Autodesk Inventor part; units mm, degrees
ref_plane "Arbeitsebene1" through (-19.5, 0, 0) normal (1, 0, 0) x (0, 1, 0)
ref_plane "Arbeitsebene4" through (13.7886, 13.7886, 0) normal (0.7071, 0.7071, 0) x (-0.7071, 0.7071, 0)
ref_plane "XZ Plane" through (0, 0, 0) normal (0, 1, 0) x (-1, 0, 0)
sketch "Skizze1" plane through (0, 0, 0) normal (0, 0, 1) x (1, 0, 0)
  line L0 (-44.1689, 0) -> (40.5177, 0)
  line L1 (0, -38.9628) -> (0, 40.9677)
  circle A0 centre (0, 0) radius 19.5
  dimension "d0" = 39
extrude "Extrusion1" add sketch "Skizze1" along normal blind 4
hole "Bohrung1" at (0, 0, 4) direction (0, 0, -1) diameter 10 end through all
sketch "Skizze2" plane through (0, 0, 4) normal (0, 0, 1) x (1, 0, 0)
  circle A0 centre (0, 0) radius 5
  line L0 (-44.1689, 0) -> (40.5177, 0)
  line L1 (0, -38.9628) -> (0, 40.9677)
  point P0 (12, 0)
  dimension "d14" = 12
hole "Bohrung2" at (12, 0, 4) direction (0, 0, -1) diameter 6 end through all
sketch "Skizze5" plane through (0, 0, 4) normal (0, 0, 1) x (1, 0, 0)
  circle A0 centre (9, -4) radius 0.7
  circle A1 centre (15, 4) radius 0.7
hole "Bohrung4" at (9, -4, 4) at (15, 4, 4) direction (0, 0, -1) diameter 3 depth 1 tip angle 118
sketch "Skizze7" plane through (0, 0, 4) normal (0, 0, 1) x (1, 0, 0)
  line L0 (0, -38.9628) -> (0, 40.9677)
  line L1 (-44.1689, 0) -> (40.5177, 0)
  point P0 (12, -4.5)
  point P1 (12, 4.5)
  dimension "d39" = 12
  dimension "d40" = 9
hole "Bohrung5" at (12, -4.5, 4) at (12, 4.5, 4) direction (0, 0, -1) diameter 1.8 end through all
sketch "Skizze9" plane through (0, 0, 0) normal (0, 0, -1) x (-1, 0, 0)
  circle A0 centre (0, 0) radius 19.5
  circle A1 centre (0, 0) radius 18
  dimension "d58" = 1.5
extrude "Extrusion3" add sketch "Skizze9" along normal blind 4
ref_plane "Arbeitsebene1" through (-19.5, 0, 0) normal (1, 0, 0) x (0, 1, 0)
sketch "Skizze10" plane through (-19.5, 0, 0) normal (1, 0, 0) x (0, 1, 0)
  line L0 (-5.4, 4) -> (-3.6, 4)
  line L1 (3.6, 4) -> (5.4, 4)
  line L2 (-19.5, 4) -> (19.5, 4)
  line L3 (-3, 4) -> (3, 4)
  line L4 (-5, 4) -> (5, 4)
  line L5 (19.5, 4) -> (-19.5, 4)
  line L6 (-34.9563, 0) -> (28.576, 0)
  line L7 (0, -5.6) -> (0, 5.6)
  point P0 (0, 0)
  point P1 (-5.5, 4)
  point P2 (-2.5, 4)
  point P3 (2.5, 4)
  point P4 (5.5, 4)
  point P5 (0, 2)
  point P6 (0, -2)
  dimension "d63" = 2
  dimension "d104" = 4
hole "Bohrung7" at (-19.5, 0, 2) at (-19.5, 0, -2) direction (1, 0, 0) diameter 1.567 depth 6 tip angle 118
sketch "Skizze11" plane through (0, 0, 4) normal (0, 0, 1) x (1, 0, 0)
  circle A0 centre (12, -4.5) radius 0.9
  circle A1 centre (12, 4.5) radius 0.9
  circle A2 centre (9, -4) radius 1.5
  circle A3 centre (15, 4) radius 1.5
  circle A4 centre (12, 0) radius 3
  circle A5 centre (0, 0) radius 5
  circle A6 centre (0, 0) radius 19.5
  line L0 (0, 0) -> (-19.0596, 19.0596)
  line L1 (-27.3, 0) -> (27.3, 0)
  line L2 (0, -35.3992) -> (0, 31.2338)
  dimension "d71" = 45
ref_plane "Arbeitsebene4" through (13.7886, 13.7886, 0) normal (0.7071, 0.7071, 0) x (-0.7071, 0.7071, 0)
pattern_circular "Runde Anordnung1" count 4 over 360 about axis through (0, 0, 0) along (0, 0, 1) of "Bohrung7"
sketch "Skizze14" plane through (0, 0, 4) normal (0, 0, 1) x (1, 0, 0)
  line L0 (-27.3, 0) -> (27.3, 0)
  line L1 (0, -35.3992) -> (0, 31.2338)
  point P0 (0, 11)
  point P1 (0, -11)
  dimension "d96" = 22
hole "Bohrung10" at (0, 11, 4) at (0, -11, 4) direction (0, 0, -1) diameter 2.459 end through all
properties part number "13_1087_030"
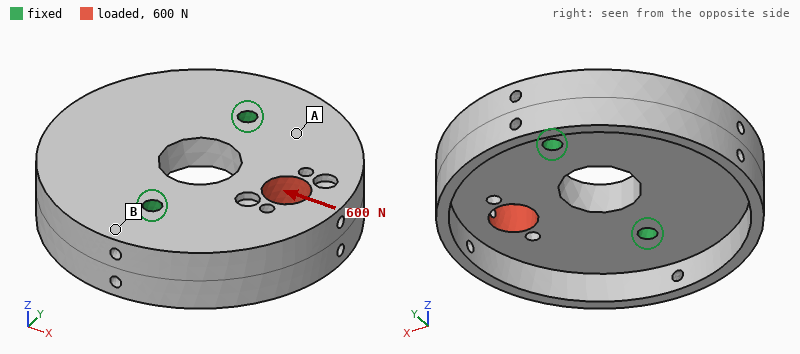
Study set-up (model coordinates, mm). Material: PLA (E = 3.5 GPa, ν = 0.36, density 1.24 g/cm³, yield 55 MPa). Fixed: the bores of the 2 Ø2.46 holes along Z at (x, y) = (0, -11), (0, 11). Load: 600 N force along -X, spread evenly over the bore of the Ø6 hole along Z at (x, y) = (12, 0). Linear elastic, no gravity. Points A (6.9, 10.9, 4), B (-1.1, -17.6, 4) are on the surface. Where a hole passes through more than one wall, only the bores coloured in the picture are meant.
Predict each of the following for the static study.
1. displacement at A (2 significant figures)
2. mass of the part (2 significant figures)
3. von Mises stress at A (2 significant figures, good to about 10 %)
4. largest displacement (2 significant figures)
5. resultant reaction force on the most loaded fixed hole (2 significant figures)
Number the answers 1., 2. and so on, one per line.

1. 12 µm
2. 6.1 g
3. 5.2 MPa
4. 72 µm
5. 330 N
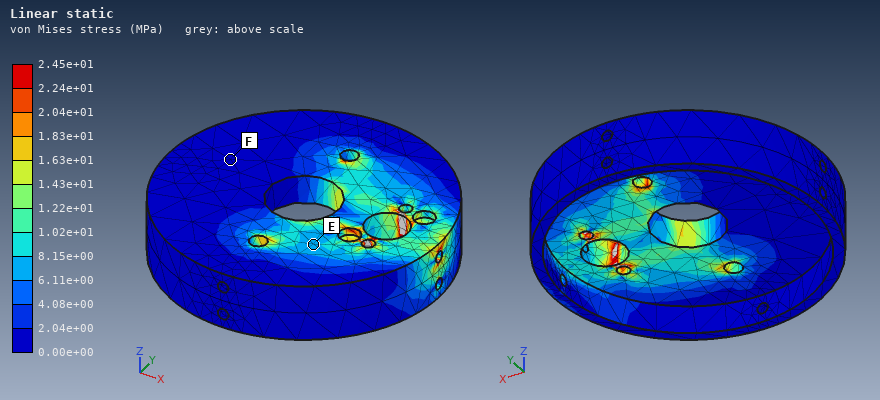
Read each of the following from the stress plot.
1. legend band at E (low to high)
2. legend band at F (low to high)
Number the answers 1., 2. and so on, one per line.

1. 6.11e+00 to 8.15e+00 MPa
2. 0.00e+00 to 2.04e+00 MPa
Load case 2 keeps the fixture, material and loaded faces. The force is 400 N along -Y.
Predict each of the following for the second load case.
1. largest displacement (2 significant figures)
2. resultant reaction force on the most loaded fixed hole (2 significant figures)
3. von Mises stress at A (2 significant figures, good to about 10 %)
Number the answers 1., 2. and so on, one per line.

1. 85 µm
2. 280 N
3. 3.6 MPa
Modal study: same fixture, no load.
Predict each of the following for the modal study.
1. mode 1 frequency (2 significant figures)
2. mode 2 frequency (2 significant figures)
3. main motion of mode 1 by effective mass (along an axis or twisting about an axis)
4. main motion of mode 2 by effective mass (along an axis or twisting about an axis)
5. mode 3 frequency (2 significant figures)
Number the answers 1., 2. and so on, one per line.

1. 2500 Hz
2. 3400 Hz
3. twisting about Y
4. along Z
5. 5200 Hz
